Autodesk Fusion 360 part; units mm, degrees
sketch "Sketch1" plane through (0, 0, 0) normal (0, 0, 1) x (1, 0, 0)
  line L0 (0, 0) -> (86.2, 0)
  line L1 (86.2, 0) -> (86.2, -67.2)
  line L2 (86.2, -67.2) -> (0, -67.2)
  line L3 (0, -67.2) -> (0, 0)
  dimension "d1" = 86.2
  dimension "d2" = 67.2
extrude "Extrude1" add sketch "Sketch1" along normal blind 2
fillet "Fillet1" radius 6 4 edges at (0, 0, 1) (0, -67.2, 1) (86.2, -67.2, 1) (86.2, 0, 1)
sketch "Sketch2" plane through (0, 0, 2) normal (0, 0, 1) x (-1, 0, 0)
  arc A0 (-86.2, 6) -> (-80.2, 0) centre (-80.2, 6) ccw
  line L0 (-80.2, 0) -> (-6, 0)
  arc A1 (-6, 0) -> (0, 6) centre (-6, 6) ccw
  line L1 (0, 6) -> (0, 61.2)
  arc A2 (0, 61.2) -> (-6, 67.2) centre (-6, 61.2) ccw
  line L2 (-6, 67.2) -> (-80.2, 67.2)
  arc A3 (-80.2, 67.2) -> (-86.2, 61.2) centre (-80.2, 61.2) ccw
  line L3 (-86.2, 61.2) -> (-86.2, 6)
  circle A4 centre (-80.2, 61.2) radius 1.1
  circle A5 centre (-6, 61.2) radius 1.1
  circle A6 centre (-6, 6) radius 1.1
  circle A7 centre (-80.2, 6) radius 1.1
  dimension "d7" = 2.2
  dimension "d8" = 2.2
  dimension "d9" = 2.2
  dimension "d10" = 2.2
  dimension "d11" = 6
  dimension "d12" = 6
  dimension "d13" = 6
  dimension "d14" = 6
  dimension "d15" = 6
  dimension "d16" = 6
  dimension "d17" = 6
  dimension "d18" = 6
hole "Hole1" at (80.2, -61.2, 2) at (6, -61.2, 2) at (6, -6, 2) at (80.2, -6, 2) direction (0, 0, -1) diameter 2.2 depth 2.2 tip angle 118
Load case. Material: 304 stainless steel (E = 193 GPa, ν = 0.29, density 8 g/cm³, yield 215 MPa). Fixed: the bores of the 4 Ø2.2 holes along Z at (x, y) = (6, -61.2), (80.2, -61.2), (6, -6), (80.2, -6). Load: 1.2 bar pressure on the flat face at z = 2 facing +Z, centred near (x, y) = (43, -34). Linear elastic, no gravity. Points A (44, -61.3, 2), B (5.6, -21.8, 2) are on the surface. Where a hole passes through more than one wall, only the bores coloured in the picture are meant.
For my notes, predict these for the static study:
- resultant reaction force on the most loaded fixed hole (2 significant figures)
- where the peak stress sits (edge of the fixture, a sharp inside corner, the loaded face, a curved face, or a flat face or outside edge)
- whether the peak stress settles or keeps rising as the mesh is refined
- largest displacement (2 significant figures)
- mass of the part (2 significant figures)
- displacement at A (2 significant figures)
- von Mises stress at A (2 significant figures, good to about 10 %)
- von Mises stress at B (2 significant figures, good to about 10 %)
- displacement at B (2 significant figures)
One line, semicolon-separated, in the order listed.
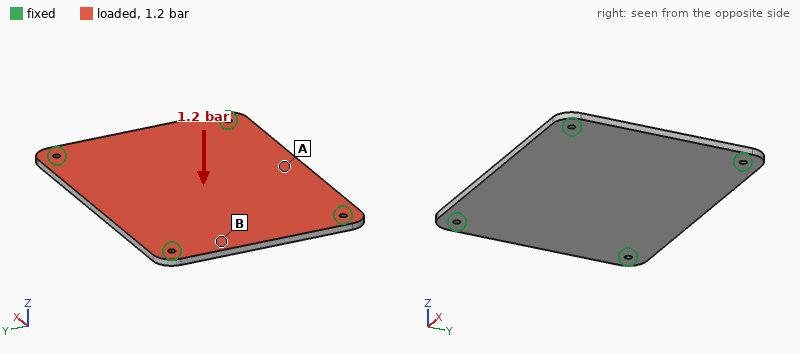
170 N; edge of the fixture; keeps rising; 0.14 mm; 92 g; 0.11 mm; 54 MPa; 25 MPa; 0.026 mm
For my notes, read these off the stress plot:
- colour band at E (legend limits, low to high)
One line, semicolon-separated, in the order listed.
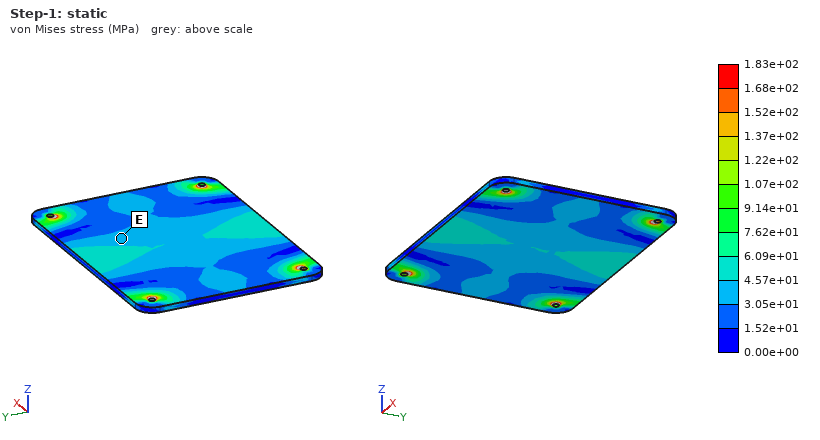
3.05e+01 to 4.57e+01 MPa
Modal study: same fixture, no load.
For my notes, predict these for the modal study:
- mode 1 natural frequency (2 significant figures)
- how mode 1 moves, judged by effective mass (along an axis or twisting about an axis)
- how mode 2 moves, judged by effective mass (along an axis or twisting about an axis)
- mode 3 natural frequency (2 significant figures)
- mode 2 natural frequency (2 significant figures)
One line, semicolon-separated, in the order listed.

1400 Hz; along Z; twisting about X; 3100 Hz; 2200 Hz
